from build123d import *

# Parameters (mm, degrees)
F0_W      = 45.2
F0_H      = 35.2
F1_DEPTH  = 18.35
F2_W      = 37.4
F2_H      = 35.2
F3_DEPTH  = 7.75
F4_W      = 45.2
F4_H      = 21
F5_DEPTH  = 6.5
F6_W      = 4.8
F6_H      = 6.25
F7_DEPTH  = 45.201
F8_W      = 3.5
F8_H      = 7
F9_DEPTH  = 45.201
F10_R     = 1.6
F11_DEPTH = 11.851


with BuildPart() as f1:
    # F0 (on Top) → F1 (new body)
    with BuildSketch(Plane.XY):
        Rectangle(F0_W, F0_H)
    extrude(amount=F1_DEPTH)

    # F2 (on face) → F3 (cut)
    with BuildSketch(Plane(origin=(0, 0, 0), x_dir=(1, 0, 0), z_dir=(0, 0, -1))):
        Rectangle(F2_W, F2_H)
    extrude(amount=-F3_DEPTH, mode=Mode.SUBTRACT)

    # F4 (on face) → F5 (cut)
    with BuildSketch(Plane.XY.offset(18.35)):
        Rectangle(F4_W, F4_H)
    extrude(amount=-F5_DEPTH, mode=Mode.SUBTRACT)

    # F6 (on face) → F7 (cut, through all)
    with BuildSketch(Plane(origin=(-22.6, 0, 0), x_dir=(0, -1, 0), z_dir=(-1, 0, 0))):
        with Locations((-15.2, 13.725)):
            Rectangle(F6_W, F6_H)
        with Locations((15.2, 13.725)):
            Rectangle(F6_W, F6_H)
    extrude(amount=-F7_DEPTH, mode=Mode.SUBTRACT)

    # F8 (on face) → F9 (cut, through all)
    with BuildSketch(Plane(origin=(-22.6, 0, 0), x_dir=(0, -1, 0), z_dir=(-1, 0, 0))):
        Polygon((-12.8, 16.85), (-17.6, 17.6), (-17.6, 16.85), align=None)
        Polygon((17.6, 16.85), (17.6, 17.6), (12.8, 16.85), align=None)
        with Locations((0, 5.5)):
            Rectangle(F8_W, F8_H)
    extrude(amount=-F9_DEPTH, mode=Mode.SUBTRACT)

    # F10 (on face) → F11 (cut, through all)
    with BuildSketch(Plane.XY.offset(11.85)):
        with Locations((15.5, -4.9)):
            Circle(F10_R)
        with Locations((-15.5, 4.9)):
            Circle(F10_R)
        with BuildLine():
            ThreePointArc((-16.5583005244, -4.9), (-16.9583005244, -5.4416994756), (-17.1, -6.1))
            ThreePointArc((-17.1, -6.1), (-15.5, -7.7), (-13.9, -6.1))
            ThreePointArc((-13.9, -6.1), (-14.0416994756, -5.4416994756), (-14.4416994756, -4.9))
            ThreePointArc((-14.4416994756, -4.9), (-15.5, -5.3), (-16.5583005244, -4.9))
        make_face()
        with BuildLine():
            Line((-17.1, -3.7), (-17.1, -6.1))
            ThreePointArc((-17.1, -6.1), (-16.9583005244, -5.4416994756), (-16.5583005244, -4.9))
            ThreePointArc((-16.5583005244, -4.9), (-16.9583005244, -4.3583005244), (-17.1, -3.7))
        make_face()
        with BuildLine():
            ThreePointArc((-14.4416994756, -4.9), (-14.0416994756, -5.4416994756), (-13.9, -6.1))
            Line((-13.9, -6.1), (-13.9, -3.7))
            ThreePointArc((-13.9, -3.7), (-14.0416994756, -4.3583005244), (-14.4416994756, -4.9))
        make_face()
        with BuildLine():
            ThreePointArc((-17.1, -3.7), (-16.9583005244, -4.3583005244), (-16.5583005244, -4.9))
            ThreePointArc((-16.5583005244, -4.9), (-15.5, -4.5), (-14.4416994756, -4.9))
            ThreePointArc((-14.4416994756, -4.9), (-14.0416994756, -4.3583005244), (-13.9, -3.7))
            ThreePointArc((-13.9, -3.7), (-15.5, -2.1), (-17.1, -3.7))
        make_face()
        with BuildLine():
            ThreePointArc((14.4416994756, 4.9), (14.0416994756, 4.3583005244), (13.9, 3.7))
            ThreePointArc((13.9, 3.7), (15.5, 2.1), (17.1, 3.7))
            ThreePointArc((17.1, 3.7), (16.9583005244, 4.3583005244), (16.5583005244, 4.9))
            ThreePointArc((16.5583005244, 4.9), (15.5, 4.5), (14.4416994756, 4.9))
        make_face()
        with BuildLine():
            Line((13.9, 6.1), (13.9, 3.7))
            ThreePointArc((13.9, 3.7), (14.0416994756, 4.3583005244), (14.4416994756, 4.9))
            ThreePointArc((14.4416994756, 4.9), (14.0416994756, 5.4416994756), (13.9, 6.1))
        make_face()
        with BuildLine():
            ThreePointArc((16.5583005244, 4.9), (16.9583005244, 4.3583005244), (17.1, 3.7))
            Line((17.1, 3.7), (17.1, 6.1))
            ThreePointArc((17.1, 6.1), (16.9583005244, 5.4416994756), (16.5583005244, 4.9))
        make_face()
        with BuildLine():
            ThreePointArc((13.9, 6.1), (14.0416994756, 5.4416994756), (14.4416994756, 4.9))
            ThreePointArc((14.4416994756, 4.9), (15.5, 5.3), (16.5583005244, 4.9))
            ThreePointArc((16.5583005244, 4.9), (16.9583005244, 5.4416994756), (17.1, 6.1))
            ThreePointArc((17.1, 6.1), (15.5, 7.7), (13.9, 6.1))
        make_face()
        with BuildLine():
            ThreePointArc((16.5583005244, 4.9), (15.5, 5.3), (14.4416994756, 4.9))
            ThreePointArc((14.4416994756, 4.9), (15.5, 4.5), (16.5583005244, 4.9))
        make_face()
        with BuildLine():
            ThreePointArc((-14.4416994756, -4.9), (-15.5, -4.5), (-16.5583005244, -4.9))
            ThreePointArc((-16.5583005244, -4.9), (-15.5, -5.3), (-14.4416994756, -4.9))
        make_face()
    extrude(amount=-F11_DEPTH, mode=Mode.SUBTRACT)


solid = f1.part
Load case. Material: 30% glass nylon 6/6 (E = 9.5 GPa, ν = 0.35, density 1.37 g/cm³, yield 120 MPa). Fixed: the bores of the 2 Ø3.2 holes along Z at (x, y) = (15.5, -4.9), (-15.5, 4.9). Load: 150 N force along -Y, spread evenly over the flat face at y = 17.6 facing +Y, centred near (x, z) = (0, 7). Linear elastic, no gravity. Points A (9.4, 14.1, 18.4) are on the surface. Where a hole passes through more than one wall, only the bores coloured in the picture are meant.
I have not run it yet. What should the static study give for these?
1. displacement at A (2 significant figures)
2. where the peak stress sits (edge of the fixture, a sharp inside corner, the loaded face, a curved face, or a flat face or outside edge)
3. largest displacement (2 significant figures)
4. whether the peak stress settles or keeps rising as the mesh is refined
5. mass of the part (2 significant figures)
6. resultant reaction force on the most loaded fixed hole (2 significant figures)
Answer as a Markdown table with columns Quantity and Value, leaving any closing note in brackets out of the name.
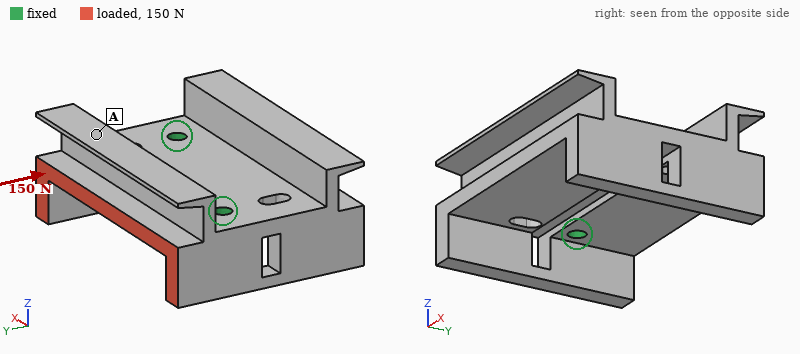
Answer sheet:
| Quantity | Value |
|---|---|
| displacement at A | 11 µm |
| where the peak stress sits | edge of the fixture |
| largest displacement | 19 µm |
| whether the peak stress settles or keeps rising as the mesh is refined | keeps rising |
| mass of the part | 13 g |
| resultant reaction force on the most loaded fixed hole | 76 N |
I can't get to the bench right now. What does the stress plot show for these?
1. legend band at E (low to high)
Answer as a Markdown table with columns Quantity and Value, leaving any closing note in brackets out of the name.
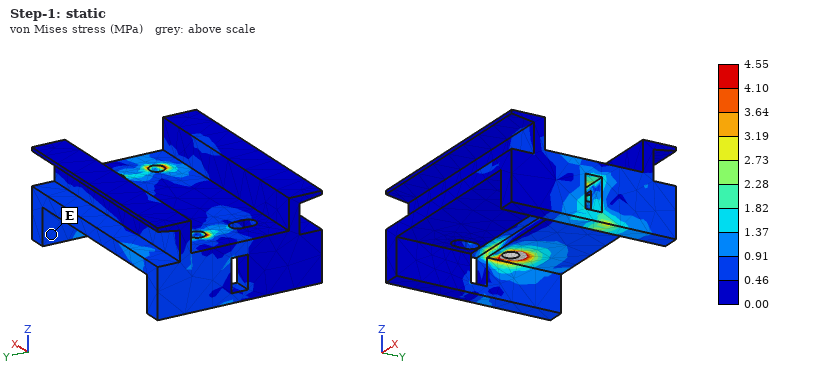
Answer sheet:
| Quantity | Value |
|---|---|
| legend band at E | 0.46 to 0.91 MPa |
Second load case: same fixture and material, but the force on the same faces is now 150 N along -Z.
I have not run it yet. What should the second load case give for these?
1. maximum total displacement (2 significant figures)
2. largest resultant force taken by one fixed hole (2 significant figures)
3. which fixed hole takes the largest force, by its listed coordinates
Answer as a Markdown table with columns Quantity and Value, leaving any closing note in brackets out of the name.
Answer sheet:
| Quantity | Value |
|---|---|
| maximum total displacement | 0.16 mm |
| largest resultant force taken by one fixed hole | 100 N |
| which fixed hole takes the largest force, by its listed coordinates | (-15.5, 4.9) |
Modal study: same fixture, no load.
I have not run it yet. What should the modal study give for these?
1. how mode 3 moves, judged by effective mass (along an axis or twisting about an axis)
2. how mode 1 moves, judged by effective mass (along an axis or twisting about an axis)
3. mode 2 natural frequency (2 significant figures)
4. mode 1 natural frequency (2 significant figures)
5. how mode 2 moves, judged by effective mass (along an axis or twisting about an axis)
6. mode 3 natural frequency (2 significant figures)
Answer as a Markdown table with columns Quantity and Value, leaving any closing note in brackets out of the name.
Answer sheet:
| Quantity | Value |
|---|---|
| how mode 3 moves, judged by effective mass | along Z |
| how mode 1 moves, judged by effective mass | twisting about X |
| mode 2 natural frequency | 3500 Hz |
| mode 1 natural frequency | 2900 Hz |
| how mode 2 moves, judged by effective mass | along Z |
| mode 3 natural frequency | 7100 Hz |
